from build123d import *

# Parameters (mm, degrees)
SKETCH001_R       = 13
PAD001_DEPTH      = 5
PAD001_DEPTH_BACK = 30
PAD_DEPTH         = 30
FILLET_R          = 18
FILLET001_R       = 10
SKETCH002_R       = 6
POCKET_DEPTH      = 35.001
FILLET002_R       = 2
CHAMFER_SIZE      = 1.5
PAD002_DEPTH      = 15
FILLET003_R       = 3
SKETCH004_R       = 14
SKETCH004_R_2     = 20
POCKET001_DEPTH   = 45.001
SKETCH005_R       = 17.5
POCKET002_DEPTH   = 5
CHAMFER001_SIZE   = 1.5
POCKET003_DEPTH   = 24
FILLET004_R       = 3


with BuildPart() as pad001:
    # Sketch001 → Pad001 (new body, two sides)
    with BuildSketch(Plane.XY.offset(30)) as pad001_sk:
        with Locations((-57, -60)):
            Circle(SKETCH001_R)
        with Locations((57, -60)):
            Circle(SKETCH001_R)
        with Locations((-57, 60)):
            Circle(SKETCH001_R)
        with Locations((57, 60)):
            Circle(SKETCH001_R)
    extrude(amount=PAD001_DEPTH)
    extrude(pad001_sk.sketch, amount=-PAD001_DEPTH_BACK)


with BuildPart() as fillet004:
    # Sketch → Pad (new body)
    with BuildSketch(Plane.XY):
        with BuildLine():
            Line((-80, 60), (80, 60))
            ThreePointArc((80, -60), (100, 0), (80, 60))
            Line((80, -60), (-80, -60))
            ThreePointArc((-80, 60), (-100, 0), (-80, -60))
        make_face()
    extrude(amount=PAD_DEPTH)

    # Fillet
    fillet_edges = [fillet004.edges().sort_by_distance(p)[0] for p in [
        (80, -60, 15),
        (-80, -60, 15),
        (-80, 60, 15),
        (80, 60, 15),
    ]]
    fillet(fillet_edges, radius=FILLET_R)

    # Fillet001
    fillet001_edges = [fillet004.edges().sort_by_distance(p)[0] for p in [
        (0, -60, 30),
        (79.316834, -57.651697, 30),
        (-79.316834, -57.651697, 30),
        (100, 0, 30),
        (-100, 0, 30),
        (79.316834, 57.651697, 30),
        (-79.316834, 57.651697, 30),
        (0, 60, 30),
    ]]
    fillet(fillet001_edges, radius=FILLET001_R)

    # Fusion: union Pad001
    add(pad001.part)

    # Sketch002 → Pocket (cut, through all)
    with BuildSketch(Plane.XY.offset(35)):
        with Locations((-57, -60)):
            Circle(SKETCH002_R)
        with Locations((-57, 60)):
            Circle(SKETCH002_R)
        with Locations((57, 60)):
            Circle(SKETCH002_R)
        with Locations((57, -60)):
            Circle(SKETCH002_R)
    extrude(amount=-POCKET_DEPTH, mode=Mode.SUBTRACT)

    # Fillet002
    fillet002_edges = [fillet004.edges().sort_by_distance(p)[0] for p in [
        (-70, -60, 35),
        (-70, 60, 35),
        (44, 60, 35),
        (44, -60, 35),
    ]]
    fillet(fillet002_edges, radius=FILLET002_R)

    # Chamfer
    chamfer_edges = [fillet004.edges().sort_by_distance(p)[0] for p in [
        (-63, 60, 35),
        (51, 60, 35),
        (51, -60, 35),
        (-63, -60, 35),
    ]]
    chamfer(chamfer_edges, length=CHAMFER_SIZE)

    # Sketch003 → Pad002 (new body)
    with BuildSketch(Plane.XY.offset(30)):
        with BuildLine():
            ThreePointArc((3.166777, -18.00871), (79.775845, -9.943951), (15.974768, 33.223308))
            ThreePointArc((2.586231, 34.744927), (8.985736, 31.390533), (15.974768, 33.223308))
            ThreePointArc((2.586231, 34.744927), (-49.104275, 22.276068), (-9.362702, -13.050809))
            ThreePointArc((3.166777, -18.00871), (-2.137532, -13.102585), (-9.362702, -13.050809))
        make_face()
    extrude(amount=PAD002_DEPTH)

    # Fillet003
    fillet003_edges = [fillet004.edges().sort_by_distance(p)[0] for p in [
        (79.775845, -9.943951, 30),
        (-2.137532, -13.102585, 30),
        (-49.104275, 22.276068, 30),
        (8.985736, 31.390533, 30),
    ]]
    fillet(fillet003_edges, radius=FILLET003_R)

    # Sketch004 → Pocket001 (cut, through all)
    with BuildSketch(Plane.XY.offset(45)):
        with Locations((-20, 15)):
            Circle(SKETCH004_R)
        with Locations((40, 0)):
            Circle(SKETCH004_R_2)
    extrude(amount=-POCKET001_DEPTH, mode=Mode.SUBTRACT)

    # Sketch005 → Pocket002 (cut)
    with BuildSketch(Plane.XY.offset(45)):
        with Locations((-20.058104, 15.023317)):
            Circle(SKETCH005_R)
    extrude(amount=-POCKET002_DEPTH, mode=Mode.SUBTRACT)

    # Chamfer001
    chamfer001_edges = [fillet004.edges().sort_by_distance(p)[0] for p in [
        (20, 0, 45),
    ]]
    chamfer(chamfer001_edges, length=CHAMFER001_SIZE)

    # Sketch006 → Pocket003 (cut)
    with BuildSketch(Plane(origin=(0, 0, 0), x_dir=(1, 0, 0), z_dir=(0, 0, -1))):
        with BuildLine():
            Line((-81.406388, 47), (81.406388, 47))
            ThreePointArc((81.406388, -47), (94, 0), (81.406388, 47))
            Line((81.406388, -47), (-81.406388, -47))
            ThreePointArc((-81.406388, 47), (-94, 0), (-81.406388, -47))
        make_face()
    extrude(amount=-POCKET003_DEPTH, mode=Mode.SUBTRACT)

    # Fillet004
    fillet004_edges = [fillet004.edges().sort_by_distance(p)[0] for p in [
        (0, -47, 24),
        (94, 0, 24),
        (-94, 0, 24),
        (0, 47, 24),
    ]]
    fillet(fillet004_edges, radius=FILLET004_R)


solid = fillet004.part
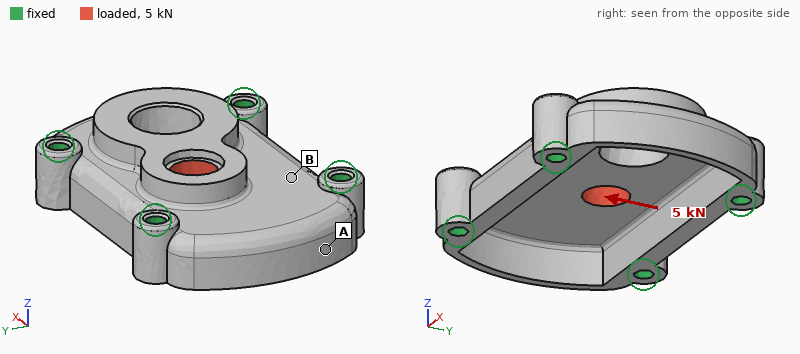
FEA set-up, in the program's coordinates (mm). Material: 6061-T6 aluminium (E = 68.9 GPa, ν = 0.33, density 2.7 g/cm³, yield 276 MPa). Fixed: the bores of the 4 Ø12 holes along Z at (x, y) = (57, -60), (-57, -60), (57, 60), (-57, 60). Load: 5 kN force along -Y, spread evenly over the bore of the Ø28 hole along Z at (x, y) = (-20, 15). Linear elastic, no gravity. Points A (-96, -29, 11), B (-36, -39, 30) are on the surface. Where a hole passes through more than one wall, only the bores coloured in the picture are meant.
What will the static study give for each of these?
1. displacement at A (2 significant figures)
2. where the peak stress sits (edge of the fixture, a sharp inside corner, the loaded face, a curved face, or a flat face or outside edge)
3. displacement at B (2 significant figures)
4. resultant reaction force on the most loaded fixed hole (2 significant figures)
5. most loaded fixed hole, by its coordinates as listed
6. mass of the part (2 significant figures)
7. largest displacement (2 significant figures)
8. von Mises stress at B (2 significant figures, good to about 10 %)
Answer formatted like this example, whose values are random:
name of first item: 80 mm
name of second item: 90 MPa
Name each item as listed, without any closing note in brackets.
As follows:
displacement at A: 1.3 µm
where the peak stress sits: a curved face
displacement at B: 2.1 µm
resultant reaction force on the most loaded fixed hole: 1.9 kN
most loaded fixed hole, by its coordinates as listed: (-57, 60)
mass of the part: 980 g
largest displacement: 7.8 µm
von Mises stress at B: 4.7 MPa
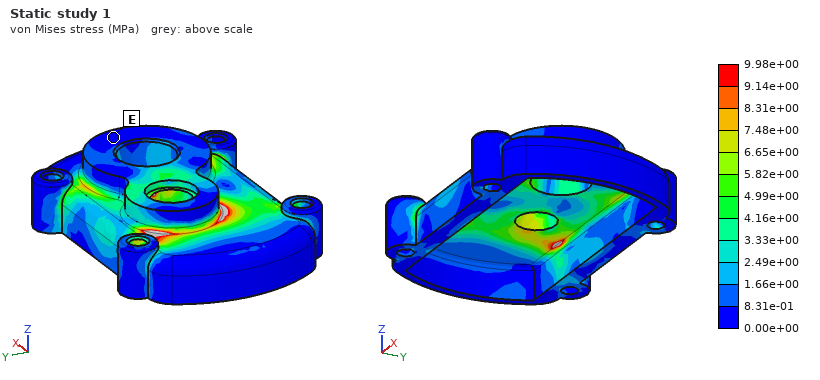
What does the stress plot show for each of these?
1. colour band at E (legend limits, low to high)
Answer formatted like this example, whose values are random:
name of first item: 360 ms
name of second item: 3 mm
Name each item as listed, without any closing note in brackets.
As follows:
colour band at E: 0.00e+00 to 8.31e-01 MPa
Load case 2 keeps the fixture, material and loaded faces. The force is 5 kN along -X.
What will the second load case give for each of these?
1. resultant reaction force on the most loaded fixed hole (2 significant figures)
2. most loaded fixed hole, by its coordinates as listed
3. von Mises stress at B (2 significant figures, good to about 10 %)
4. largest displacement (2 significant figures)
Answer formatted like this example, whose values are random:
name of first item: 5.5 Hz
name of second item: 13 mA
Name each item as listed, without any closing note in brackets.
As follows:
resultant reaction force on the most loaded fixed hole: 1.8 kN
most loaded fixed hole, by its coordinates as listed: (-57, 60)
von Mises stress at B: 3.2 MPa
largest displacement: 6.2 µm
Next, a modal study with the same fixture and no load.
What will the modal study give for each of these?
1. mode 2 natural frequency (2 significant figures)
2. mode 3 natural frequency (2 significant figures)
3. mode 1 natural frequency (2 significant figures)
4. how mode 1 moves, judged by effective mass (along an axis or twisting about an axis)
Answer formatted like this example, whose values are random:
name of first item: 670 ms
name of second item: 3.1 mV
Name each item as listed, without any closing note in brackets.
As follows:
mode 2 natural frequency: 5200 Hz
mode 3 natural frequency: 5400 Hz
mode 1 natural frequency: 4000 Hz
how mode 1 moves, judged by effective mass: along Z
